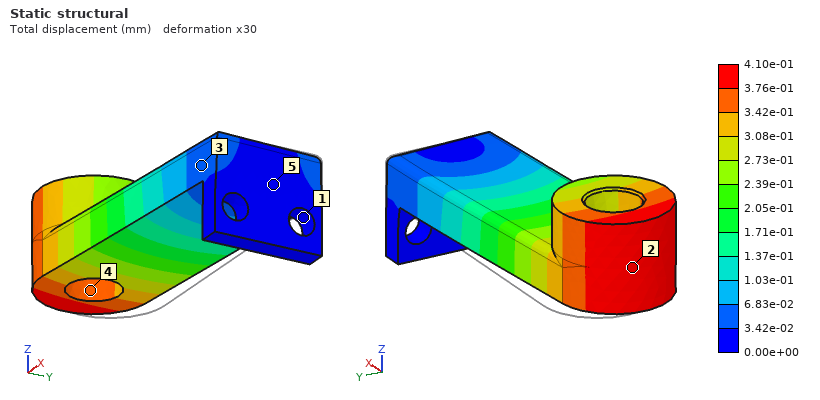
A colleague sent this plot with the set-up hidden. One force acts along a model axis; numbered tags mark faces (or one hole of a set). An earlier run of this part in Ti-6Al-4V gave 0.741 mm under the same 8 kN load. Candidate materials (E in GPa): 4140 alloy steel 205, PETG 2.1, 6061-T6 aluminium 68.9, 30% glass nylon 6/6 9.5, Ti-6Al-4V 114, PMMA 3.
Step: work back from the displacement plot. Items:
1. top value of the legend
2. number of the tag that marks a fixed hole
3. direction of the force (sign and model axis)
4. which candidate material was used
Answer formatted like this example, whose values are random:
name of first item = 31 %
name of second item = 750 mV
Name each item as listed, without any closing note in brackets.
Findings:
top value of the legend = 4.10e-01 mm
number of the tag that marks a fixed hole = 1
direction of the force = -Y
which candidate material was used = 4140 alloy steel
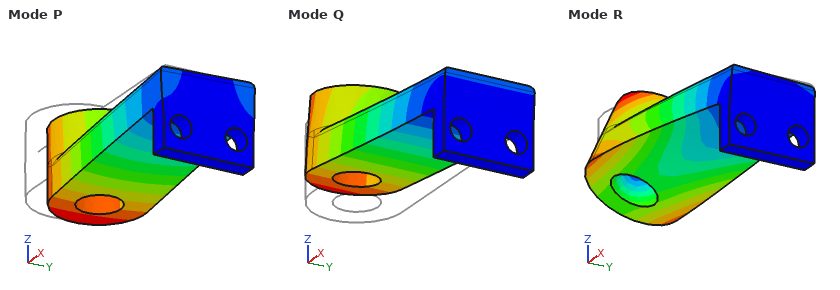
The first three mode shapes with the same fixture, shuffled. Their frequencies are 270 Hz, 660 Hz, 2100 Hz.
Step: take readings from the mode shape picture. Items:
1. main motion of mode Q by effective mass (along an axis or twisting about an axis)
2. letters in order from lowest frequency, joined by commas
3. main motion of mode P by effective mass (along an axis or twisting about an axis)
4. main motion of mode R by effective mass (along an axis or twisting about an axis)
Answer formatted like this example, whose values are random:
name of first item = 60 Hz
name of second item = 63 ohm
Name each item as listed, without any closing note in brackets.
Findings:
main motion of mode Q by effective mass = along Z
letters in order from lowest frequency, joined by commas = Q, P, R
main motion of mode P by effective mass = along Y
main motion of mode R by effective mass = twisting about X
